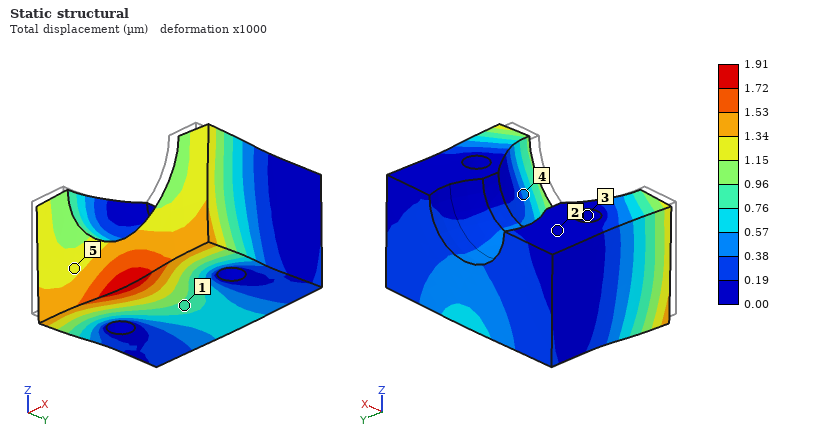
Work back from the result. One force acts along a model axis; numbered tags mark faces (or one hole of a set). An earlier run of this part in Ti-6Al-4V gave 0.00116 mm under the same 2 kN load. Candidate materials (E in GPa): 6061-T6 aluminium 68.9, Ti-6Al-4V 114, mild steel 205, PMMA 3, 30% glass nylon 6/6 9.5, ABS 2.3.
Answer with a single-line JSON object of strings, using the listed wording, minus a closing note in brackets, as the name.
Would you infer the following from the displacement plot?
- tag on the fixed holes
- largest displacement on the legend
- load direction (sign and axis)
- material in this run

{"tag on the fixed holes": "3", "largest displacement on the legend": "1.91 µm", "load direction": "+Y", "material in this run": "6061-T6 aluminium"}
